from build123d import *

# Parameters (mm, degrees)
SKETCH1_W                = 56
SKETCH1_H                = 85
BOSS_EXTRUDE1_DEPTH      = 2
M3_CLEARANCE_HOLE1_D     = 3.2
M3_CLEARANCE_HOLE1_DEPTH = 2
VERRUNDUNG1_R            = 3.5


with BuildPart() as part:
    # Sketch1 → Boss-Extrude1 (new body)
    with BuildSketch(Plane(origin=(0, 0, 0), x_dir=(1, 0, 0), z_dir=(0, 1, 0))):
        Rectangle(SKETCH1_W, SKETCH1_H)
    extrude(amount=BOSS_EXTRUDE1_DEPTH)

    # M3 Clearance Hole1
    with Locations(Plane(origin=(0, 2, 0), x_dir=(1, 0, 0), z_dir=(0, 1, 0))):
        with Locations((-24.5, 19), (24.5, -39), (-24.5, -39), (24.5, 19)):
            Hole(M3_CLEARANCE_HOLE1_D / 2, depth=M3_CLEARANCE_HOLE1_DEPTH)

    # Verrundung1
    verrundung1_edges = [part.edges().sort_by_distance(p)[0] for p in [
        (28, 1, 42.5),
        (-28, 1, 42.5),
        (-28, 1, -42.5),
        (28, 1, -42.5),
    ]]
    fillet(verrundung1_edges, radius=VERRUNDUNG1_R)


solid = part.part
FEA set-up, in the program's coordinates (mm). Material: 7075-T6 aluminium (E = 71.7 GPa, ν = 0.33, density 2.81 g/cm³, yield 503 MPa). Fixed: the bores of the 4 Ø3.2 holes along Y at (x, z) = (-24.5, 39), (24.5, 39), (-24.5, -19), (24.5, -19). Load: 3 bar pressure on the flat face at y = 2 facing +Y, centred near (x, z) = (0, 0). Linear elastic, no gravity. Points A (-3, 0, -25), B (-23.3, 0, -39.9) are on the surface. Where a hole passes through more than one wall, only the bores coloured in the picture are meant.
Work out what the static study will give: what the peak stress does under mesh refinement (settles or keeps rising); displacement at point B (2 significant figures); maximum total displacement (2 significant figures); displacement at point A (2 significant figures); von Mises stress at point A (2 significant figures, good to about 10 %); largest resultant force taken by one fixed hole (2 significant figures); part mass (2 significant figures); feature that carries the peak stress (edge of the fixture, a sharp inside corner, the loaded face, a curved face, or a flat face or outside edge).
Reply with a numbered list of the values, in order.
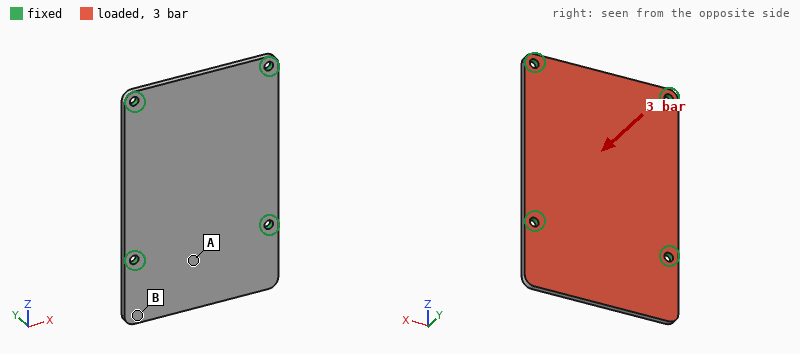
1. keeps rising
2. 0.20 mm
3. 0.37 mm
4. 0.19 mm
5. 82 MPa
6. 450 N
7. 27 g
8. edge of the fixture
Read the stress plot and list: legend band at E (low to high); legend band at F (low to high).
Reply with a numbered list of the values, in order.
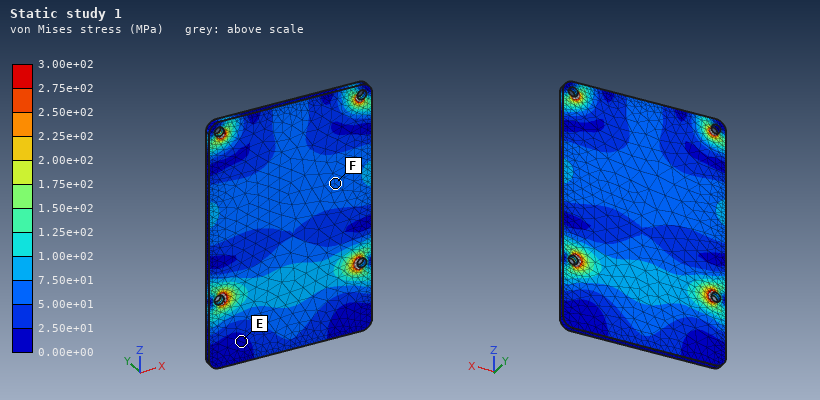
1. 0.00e+00 to 2.50e+01 MPa
2. 5.00e+01 to 7.50e+01 MPa
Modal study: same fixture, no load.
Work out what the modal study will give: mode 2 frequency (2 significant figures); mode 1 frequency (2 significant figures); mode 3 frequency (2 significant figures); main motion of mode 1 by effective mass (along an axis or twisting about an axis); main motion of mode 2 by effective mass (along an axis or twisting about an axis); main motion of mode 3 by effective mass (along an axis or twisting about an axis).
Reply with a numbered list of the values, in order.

1. 2500 Hz
2. 2100 Hz
3. 3700 Hz
4. twisting about X
5. along Y
6. twisting about Z
